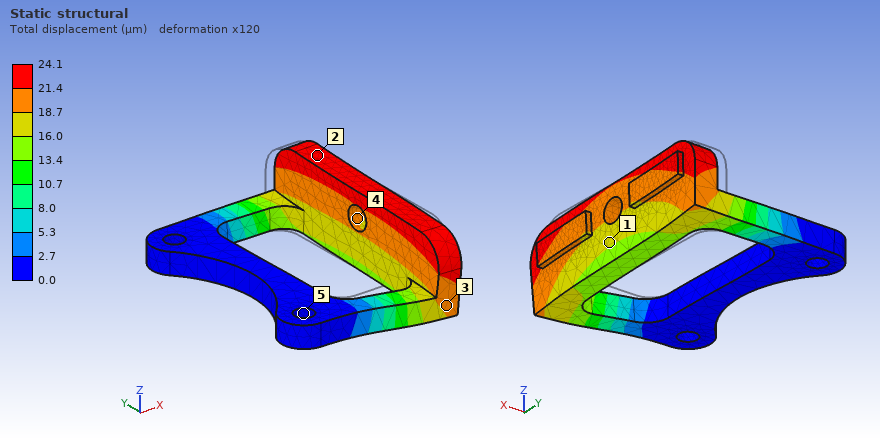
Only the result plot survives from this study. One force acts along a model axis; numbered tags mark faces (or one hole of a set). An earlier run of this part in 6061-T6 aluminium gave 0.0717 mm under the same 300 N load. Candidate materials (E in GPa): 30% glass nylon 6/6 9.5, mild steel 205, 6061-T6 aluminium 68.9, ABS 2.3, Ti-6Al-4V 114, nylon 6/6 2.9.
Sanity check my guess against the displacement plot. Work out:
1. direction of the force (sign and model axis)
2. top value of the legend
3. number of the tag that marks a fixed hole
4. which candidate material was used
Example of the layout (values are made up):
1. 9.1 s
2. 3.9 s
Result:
1. -Y
2. 24.1 µm
3. 5
4. mild steel
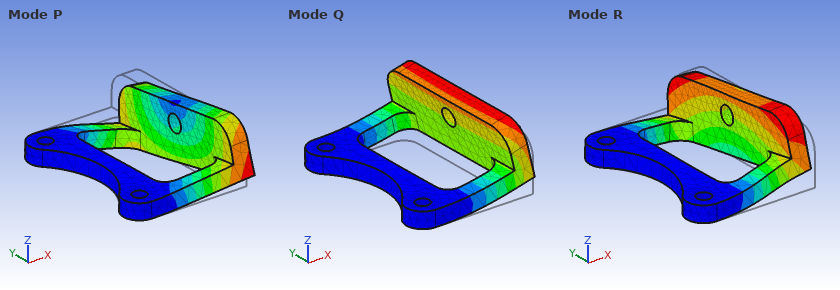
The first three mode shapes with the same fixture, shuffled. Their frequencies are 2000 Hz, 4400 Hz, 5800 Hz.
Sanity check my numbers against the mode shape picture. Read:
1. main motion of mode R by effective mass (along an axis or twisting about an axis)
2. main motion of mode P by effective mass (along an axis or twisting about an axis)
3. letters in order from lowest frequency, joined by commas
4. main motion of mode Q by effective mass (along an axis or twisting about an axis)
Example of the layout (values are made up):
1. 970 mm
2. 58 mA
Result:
1. along Y
2. along Y
3. Q, R, P
4. along Z
